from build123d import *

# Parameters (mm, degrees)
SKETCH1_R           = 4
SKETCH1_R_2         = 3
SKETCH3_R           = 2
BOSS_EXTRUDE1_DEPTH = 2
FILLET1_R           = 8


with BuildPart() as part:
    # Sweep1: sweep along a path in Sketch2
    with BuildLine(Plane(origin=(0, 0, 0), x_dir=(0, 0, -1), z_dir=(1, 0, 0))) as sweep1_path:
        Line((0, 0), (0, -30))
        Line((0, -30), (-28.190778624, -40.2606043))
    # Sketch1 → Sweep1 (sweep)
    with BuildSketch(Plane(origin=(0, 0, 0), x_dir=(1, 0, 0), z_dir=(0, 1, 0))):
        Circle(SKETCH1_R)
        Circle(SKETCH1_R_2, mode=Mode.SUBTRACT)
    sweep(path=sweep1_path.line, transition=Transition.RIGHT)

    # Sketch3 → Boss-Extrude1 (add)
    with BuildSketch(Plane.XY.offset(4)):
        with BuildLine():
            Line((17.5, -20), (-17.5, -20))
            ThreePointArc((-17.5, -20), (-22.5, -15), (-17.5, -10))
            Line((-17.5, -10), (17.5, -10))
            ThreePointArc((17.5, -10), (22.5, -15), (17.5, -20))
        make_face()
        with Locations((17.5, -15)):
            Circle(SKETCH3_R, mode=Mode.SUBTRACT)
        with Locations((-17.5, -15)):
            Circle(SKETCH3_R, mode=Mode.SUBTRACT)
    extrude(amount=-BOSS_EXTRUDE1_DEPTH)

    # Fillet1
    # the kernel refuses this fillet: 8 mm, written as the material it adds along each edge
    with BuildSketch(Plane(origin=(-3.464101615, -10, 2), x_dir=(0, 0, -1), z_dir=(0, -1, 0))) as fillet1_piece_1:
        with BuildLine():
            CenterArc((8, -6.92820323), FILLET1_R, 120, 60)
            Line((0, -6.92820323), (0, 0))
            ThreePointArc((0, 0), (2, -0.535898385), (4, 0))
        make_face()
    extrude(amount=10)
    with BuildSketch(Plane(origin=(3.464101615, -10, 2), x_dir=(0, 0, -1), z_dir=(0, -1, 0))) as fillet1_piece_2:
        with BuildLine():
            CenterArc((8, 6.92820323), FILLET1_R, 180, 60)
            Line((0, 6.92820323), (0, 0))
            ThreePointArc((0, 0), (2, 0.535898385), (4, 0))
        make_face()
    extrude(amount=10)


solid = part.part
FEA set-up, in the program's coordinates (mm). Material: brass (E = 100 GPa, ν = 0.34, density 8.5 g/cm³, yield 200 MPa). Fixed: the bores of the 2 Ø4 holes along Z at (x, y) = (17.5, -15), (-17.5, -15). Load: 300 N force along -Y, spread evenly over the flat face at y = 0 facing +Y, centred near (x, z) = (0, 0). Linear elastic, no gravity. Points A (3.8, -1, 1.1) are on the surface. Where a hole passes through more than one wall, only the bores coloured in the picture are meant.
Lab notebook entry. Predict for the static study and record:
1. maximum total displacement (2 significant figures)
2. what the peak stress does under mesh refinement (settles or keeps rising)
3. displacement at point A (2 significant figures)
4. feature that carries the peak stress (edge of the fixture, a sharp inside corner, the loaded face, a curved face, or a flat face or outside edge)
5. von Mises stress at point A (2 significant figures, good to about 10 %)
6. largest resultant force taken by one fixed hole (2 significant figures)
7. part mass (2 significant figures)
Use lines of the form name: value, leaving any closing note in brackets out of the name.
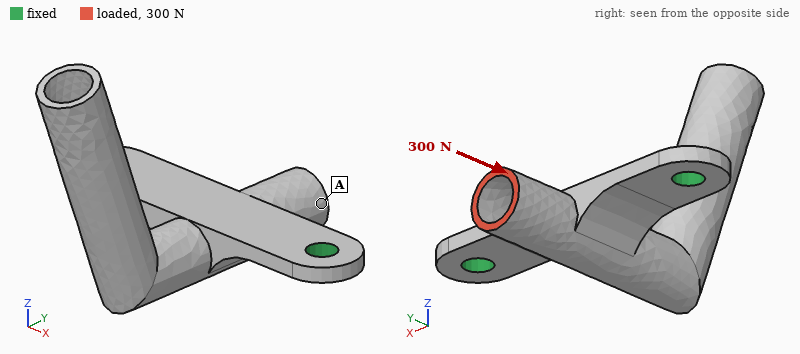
maximum total displacement: 0.13 mm
what the peak stress does under mesh refinement: keeps rising
displacement at point A: 0.053 mm
feature that carries the peak stress: edge of the fixture
von Mises stress at point A: 13 MPa
largest resultant force taken by one fixed hole: 150 N
part mass: 19 g
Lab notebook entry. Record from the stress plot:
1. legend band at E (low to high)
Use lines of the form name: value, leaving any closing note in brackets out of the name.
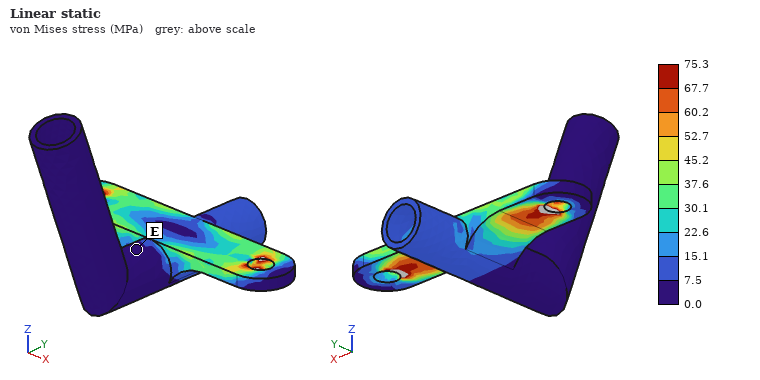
legend band at E: 0.0 to 7.5 MPa
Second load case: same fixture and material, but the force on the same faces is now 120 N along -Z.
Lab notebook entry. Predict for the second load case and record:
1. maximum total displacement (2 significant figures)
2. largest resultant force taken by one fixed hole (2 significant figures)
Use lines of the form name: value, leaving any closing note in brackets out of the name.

maximum total displacement: 0.26 mm
largest resultant force taken by one fixed hole: 86 N
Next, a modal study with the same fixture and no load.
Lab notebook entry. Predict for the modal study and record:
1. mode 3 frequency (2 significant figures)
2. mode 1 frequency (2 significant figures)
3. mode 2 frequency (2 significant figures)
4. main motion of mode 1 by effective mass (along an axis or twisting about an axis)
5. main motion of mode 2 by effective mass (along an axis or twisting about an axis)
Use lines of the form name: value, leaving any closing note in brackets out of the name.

mode 3 frequency: 4200 Hz
mode 1 frequency: 1100 Hz
mode 2 frequency: 2200 Hz
main motion of mode 1 by effective mass: along Z
main motion of mode 2 by effective mass: along X
